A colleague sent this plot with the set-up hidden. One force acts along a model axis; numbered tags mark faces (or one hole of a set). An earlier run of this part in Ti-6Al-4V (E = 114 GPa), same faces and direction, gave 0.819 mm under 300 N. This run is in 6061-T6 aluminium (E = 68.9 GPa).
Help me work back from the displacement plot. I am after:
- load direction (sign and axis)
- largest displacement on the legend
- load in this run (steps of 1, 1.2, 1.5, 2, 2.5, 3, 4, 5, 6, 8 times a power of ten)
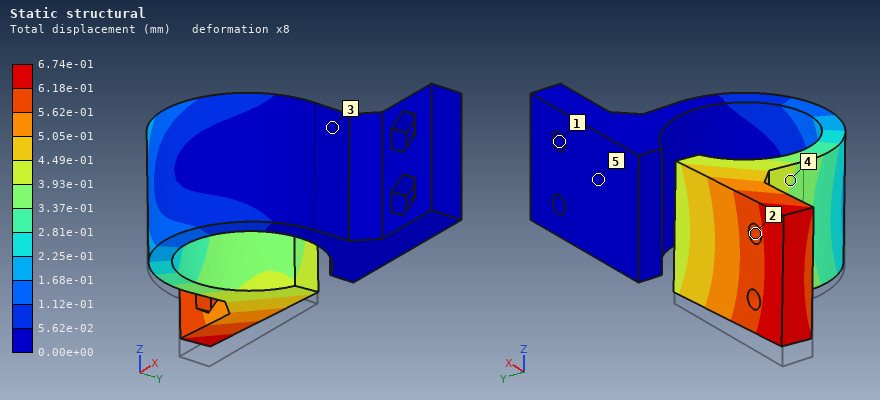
+Z
6.74e-01 mm
150 N
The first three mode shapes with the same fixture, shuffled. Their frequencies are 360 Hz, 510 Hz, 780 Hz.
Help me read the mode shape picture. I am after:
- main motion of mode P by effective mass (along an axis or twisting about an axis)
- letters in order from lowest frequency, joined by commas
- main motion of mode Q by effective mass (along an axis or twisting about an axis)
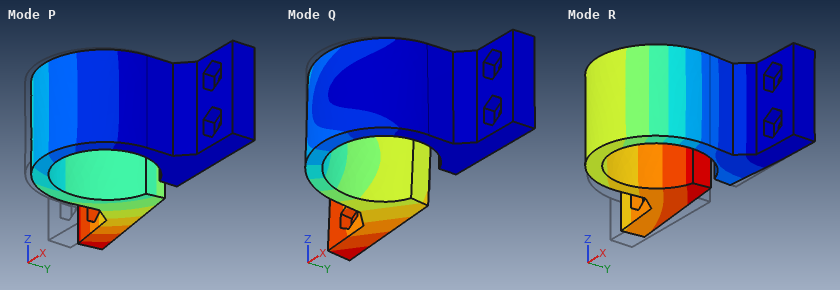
along Y
P, Q, R
along Z
